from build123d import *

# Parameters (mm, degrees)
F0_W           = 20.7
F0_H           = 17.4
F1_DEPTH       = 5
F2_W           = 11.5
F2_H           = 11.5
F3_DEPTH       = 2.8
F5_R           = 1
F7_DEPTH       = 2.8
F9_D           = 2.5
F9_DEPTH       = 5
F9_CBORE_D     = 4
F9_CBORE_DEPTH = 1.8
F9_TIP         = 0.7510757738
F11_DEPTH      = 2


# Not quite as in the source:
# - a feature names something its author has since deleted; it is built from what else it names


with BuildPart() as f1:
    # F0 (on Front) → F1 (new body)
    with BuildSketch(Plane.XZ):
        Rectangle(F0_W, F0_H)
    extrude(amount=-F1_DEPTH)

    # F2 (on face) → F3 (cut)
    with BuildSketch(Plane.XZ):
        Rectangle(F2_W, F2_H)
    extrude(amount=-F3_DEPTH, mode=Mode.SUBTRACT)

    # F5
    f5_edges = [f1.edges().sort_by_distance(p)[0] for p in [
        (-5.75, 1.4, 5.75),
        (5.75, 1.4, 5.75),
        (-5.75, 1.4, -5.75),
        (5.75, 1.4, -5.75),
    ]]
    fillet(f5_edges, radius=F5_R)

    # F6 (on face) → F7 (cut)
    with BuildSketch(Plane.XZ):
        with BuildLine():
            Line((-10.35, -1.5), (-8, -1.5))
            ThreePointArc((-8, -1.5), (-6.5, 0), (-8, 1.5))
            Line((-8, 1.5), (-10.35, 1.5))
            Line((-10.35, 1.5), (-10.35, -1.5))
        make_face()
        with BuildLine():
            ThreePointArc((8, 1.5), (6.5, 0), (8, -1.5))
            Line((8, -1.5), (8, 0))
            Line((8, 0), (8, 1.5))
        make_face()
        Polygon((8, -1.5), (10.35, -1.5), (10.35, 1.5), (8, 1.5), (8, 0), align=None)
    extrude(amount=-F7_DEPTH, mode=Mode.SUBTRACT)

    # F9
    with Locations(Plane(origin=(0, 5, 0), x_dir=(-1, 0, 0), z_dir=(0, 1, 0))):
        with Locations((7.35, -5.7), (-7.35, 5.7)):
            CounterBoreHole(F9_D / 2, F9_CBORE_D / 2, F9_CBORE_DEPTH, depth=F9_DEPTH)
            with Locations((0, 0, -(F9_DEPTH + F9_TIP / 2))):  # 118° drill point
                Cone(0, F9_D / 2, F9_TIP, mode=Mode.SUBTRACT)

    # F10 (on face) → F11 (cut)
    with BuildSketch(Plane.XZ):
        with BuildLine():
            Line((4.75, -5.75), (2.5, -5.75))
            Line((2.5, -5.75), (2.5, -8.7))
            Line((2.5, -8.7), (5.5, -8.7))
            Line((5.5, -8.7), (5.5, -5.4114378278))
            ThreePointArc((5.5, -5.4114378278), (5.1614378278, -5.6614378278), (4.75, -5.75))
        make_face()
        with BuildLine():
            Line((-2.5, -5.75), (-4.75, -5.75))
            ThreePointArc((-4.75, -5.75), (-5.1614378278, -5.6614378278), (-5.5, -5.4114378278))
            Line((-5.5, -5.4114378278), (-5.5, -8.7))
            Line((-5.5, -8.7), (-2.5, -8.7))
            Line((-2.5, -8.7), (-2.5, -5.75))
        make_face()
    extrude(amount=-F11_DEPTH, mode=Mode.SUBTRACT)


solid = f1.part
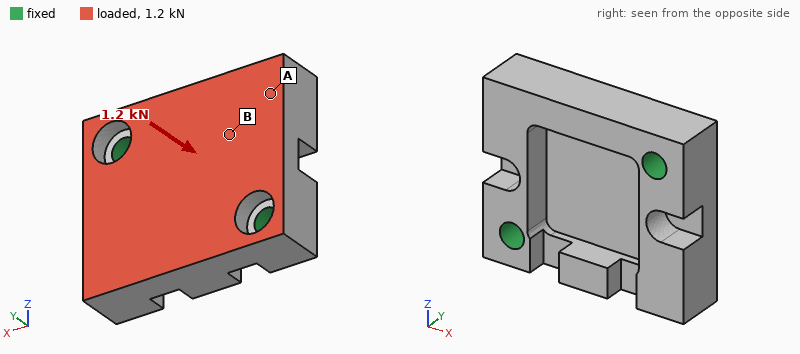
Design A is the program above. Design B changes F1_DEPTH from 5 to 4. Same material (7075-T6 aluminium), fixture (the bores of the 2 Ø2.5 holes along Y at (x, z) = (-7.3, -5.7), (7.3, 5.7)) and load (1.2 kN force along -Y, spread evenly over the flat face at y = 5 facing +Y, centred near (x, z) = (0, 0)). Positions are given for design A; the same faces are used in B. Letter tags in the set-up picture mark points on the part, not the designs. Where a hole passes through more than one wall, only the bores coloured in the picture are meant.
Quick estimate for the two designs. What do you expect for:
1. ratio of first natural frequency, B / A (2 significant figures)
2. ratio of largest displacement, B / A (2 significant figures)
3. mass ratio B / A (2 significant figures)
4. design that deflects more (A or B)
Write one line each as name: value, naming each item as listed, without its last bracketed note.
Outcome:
ratio of first natural frequency, B / A: 0.86
ratio of largest displacement, B / A: 2.2
mass ratio B / A: 0.73
design that deflects more: B
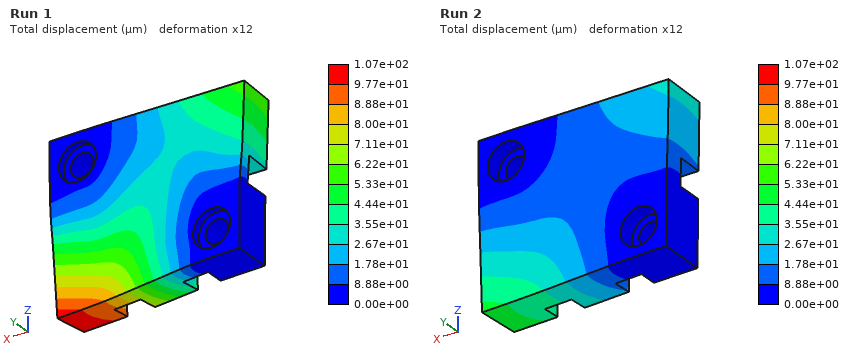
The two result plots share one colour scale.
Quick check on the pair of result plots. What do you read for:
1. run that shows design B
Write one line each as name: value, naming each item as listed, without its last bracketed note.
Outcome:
run that shows design B: Run 1
